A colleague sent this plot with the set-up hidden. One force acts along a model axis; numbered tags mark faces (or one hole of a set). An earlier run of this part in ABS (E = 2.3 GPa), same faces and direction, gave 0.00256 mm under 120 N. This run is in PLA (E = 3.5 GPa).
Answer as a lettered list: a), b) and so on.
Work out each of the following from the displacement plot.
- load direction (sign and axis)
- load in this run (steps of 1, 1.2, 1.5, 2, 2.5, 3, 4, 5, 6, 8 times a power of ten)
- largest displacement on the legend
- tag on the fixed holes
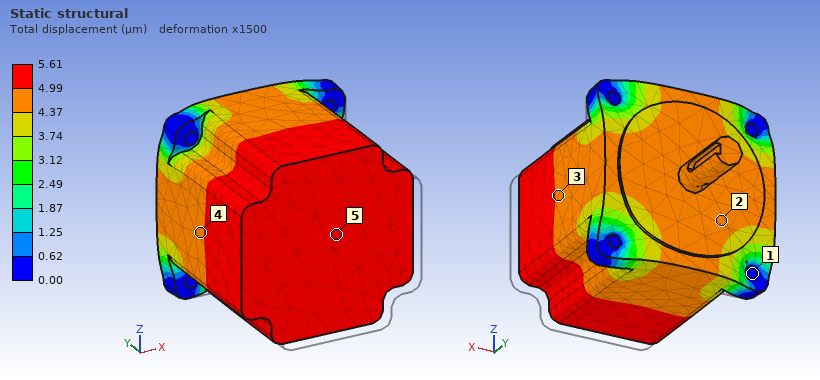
a) +Y
b) 400 N
c) 5.61 µm
d) 1
